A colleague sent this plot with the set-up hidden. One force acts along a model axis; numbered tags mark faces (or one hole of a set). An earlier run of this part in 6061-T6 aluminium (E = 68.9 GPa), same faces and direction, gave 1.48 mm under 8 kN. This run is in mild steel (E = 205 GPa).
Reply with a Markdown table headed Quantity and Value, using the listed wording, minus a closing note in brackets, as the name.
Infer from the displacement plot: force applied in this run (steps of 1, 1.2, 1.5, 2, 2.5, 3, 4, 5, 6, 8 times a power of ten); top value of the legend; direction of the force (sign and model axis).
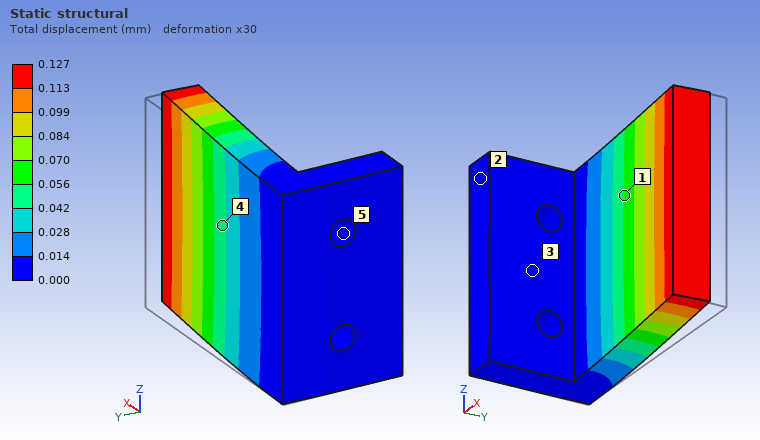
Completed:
| Quantity | Value |
|---|---|
| force applied in this run | 2 kN |
| top value of the legend | 0.127 mm |
| direction of the force | -Y |
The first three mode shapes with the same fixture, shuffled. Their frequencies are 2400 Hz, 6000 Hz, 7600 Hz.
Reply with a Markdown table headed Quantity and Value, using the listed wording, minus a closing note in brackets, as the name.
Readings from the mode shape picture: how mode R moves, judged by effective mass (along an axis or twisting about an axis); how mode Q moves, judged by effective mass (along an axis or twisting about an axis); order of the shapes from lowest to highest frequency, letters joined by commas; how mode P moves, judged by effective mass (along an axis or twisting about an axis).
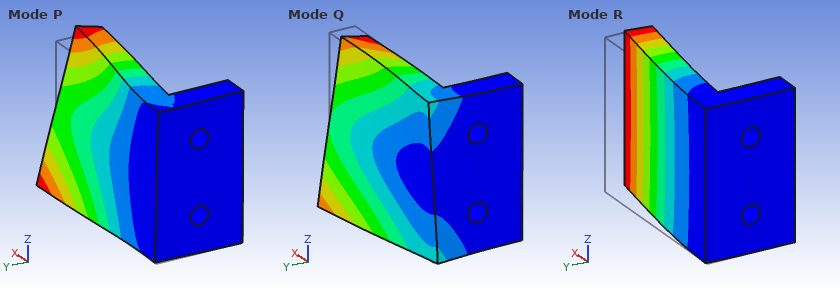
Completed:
| Quantity | Value |
|---|---|
| how mode R moves, judged by effective mass | along Y |
| how mode Q moves, judged by effective mass | along Z |
| order of the shapes from lowest to highest frequency, letters joined by commas | R, Q, P |
| how mode P moves, judged by effective mass | along Z |
